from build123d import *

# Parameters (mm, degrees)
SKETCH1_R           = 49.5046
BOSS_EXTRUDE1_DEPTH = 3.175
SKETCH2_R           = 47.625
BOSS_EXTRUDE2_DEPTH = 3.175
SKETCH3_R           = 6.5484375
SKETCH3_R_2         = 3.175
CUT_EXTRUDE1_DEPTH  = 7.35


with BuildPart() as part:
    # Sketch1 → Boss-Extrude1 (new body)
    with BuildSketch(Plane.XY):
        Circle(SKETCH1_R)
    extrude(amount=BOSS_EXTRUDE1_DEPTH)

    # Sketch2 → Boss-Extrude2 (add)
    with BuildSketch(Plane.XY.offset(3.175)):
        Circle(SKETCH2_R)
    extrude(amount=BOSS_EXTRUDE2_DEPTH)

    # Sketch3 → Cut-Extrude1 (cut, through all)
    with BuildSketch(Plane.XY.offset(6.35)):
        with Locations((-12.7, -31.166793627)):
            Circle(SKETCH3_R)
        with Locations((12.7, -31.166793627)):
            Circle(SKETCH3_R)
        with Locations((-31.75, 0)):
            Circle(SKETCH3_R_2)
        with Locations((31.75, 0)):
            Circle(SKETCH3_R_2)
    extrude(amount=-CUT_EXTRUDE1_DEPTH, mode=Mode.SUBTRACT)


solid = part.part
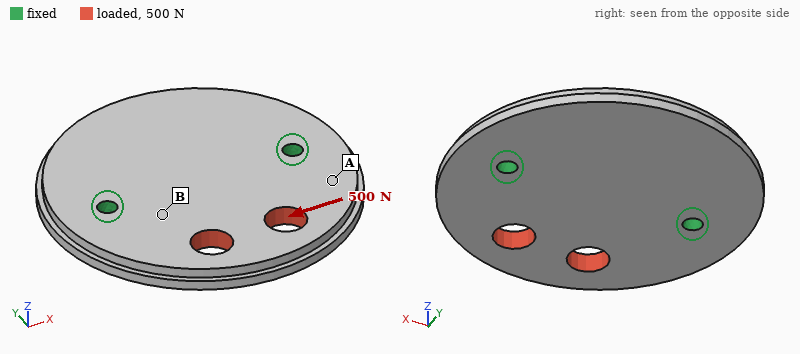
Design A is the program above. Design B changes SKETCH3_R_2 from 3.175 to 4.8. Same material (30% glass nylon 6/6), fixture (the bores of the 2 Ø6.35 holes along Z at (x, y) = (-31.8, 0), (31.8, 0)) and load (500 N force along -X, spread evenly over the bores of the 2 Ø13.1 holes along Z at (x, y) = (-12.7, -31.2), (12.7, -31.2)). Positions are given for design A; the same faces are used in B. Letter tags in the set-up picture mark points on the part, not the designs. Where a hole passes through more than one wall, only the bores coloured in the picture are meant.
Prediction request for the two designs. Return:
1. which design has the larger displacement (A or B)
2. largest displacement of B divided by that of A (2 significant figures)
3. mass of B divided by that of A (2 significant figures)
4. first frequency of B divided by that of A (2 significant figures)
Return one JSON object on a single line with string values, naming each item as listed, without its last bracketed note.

{"which design has the larger displacement": "A", "largest displacement of B divided by that of A": "0.92", "mass of B divided by that of A": "0.99", "first frequency of B divided by that of A": "1.1"}
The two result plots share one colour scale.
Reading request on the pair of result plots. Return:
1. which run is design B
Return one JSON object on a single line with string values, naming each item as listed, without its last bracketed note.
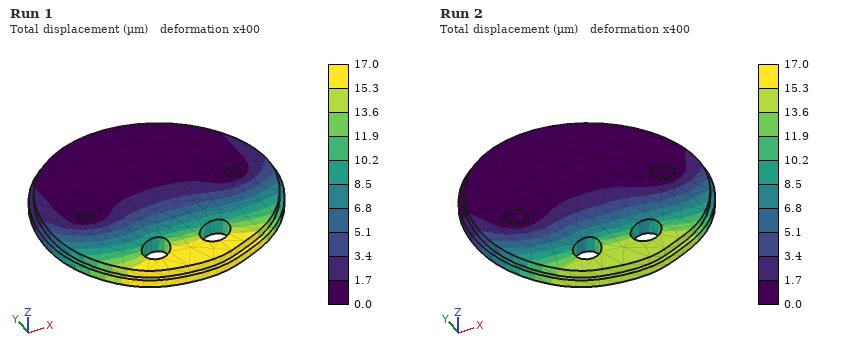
{"which run is design B": "Run 2"}
